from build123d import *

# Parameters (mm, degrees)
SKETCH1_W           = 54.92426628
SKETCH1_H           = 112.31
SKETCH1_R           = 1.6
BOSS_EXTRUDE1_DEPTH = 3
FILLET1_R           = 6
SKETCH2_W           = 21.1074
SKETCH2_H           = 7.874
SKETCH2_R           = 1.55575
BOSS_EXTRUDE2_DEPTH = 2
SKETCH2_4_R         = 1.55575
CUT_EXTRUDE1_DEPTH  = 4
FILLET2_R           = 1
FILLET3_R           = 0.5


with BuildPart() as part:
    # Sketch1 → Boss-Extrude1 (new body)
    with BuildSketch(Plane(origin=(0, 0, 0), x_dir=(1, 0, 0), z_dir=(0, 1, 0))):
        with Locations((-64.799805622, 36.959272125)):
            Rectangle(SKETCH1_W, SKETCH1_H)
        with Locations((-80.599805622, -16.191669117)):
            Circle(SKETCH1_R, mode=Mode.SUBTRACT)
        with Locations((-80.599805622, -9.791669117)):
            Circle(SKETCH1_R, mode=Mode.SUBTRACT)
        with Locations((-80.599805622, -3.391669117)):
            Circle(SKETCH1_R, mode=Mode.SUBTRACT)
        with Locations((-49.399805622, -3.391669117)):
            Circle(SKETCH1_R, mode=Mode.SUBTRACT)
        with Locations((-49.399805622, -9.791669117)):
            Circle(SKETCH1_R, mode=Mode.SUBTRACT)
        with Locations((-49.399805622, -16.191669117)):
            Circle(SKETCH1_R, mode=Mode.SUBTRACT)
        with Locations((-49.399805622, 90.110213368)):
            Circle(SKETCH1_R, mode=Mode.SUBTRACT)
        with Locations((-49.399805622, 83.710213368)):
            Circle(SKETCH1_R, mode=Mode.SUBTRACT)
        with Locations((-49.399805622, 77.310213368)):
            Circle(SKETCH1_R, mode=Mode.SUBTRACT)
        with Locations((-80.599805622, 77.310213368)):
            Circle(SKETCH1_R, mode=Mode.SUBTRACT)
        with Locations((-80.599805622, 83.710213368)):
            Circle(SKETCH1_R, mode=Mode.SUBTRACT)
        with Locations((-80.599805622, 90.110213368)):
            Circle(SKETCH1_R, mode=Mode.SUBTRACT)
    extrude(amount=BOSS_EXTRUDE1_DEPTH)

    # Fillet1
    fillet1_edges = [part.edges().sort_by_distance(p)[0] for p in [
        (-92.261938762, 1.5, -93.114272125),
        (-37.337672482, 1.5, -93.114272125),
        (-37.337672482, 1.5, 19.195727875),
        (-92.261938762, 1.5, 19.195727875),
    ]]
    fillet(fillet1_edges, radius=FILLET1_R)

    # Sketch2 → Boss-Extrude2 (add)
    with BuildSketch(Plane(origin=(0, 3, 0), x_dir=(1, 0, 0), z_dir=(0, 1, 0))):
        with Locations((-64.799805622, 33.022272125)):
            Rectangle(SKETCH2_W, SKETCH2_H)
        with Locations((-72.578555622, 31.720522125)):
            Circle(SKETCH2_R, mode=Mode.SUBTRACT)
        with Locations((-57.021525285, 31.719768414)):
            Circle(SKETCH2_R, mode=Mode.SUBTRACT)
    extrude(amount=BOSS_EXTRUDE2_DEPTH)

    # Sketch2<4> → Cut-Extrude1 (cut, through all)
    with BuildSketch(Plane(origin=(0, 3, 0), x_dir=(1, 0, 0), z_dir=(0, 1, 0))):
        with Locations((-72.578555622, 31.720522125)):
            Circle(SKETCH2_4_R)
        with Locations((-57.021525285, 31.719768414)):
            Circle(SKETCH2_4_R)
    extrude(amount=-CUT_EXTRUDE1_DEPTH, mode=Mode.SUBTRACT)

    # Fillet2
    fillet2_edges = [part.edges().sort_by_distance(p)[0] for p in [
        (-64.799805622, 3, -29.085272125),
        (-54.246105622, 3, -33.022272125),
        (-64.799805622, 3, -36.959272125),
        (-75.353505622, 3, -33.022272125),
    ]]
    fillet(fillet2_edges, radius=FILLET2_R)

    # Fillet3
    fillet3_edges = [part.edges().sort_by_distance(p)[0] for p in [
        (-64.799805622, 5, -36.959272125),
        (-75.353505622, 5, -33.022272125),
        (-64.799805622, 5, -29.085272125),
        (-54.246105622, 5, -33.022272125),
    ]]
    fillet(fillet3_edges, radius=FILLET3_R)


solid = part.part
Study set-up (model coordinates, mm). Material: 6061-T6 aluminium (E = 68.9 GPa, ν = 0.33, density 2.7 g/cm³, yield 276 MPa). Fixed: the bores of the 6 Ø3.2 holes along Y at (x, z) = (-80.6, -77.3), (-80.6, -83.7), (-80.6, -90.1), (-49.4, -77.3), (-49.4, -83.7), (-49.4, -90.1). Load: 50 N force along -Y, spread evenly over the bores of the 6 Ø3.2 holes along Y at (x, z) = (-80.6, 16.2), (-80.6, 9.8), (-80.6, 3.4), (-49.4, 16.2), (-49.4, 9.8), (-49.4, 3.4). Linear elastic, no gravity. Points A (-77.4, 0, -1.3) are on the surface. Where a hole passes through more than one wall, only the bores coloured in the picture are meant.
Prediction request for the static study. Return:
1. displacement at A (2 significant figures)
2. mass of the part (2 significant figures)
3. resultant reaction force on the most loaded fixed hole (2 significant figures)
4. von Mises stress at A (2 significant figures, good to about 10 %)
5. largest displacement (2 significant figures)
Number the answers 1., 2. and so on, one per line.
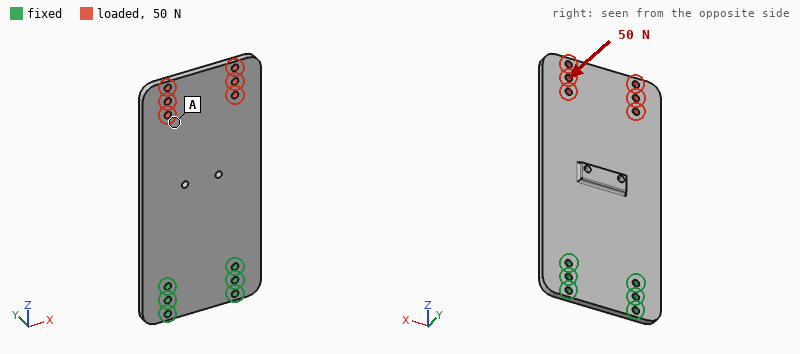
1. 1.0 mm
2. 50 g
3. 150 N
4. 7.7 MPa
5. 1.5 mm
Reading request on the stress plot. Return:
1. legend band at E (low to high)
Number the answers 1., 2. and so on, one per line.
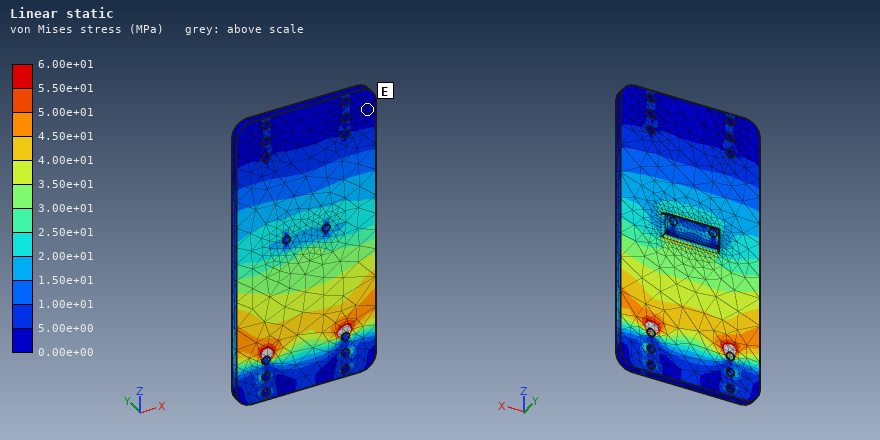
1. 0.00e+00 to 5.00e+00 MPa
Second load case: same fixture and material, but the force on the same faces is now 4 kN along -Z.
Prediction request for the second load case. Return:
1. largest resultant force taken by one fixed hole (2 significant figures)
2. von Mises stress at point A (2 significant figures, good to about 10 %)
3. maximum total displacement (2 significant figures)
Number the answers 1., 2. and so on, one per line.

1. 1.3 kN
2. 34 MPa
3. 48 µm
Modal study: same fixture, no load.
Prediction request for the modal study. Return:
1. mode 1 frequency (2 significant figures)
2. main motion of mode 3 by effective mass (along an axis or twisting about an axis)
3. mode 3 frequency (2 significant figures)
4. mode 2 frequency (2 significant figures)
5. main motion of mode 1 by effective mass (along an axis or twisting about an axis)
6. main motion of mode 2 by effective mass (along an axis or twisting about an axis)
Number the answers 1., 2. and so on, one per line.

1. 270 Hz
2. along Y
3. 1700 Hz
4. 1000 Hz
5. along Y
6. twisting about Z
